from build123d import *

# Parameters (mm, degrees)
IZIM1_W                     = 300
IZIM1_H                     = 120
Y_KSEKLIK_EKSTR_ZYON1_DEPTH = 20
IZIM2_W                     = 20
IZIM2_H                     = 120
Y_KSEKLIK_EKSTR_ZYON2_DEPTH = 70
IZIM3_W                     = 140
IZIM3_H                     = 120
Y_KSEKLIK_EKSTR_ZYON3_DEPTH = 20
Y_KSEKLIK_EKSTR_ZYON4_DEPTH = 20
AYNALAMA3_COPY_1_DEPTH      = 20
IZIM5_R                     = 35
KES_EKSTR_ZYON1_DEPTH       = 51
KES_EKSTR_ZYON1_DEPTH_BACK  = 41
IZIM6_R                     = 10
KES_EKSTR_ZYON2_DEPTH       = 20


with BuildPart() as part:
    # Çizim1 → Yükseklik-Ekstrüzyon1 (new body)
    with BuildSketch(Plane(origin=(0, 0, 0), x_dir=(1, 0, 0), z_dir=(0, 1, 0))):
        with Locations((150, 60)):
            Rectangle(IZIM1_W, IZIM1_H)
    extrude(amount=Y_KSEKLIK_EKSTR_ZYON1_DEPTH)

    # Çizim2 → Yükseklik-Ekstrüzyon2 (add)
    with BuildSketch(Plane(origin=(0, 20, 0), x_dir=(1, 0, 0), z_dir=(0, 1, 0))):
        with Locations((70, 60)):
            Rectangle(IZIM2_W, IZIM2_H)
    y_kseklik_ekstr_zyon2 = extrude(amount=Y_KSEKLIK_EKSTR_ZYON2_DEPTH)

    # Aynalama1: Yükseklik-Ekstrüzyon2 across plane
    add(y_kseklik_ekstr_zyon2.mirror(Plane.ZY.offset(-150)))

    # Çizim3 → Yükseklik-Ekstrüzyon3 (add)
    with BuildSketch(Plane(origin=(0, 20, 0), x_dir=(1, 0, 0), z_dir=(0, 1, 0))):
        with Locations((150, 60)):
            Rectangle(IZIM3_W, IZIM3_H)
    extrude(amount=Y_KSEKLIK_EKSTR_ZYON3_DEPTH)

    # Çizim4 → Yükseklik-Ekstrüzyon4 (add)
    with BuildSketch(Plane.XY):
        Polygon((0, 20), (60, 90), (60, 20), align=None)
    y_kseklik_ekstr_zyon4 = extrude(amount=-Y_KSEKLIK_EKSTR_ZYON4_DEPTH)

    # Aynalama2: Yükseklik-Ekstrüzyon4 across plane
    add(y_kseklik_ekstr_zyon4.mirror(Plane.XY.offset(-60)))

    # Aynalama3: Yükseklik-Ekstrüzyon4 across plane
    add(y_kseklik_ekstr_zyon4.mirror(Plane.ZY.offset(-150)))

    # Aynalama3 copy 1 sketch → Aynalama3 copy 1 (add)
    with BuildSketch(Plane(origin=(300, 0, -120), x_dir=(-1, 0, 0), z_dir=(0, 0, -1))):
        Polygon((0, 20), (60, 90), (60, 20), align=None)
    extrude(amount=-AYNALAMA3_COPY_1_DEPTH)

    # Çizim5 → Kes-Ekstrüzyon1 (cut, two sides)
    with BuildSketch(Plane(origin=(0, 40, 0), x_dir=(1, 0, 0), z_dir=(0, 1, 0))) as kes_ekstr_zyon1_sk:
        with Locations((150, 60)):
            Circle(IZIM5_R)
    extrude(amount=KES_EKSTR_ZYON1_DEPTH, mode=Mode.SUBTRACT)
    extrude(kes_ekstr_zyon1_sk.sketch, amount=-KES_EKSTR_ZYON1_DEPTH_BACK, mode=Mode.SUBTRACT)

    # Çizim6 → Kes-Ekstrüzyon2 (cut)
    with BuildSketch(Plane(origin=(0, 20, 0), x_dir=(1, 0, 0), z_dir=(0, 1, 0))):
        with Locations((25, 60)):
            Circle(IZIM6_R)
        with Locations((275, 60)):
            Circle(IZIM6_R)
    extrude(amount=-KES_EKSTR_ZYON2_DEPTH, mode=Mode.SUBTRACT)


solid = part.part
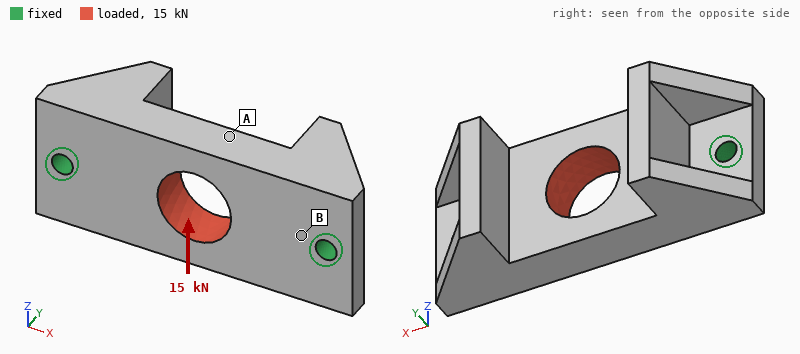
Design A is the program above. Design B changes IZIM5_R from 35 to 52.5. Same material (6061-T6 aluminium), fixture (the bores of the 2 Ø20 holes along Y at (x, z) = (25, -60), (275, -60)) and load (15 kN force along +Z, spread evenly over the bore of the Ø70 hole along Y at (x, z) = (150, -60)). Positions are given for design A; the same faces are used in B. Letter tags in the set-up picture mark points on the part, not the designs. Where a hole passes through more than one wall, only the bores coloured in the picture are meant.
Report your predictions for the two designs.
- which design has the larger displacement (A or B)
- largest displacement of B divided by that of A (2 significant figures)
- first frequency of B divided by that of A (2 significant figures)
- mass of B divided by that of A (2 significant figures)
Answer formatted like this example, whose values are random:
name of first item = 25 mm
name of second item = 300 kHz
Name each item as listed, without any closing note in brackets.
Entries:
which design has the larger displacement = B
largest displacement of B divided by that of A = 1.1
first frequency of B divided by that of A = 1.0
mass of B divided by that of A = 0.86
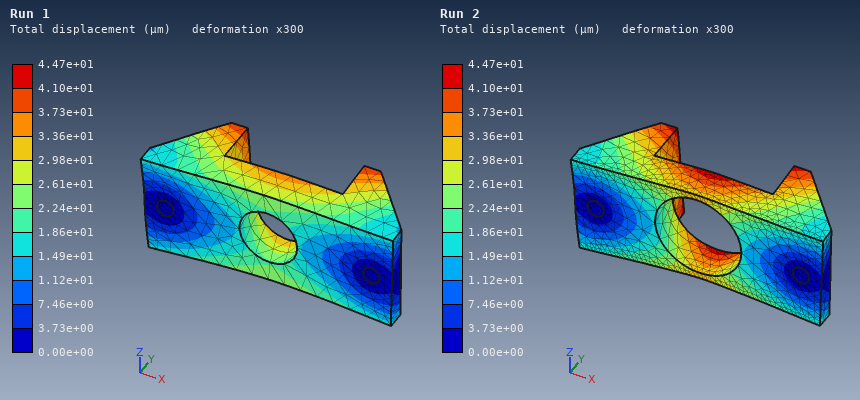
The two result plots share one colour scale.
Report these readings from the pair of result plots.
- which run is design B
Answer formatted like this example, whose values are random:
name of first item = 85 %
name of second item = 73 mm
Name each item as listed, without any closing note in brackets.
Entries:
which run is design B = Run 2
